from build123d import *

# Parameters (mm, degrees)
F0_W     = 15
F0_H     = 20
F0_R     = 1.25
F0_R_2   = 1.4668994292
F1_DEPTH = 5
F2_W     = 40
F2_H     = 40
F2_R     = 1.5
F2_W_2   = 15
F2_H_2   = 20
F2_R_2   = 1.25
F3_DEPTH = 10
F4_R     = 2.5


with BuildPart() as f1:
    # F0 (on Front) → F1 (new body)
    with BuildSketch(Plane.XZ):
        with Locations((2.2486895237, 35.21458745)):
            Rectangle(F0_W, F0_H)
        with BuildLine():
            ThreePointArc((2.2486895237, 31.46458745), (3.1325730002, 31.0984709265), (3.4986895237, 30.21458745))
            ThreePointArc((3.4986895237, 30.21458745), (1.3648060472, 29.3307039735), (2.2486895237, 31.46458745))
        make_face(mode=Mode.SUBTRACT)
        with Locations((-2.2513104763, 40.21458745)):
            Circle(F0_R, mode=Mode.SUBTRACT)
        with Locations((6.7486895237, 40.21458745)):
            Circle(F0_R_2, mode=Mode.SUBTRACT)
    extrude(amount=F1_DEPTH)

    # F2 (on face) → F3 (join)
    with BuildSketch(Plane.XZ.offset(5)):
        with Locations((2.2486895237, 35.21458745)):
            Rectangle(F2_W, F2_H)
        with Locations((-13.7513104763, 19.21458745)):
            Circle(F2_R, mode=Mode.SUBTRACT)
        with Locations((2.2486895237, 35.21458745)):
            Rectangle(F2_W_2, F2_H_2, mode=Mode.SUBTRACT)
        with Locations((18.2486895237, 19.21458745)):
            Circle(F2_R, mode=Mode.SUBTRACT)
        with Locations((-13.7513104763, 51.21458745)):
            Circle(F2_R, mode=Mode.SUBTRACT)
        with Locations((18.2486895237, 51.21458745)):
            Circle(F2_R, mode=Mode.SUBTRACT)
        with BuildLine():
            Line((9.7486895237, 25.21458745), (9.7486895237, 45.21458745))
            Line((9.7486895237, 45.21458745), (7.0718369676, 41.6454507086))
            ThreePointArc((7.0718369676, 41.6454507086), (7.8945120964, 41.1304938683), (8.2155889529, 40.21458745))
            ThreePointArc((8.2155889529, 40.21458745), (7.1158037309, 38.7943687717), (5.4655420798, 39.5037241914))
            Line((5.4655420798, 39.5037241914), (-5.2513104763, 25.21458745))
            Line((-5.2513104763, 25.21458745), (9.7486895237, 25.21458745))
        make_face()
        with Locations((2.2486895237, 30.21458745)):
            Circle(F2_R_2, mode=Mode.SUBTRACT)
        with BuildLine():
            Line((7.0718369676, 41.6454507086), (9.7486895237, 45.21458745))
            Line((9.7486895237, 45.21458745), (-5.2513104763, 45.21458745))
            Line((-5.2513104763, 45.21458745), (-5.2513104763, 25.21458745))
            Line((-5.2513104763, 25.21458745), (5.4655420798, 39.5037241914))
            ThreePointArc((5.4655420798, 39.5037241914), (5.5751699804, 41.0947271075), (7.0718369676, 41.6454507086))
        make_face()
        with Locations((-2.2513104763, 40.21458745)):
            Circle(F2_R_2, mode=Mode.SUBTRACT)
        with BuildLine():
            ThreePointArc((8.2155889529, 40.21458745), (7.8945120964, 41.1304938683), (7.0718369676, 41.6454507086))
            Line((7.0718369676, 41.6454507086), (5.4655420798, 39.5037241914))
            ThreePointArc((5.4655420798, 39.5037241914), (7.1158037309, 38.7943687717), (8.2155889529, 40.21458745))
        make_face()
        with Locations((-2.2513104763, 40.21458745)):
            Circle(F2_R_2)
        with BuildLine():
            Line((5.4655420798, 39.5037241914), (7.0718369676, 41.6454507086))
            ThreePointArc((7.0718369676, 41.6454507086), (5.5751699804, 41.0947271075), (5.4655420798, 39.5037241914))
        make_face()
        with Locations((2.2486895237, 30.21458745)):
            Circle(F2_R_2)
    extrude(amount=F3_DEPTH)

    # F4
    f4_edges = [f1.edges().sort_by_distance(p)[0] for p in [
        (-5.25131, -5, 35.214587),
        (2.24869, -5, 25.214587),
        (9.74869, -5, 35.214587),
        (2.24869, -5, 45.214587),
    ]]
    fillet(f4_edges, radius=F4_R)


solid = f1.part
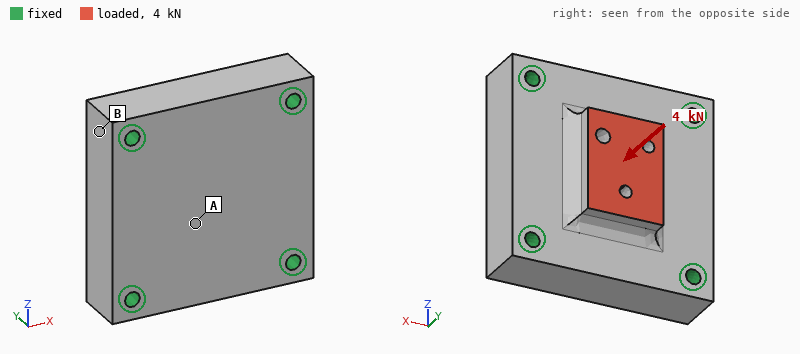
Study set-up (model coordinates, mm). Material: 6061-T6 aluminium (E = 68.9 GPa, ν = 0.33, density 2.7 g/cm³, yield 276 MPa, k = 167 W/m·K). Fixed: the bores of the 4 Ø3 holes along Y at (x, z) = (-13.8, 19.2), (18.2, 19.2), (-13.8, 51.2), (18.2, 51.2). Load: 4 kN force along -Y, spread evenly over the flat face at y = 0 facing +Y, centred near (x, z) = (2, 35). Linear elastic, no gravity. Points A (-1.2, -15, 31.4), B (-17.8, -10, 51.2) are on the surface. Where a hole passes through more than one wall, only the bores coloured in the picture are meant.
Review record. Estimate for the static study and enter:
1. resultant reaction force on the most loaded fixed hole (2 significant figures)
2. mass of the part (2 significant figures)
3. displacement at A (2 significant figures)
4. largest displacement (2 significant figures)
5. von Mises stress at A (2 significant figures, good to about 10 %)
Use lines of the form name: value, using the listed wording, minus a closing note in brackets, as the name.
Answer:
resultant reaction force on the most loaded fixed hole: 1.0 kN
mass of the part: 47 g
displacement at A: 7.9 µm
largest displacement: 9.3 µm
von Mises stress at A: 17 MPa
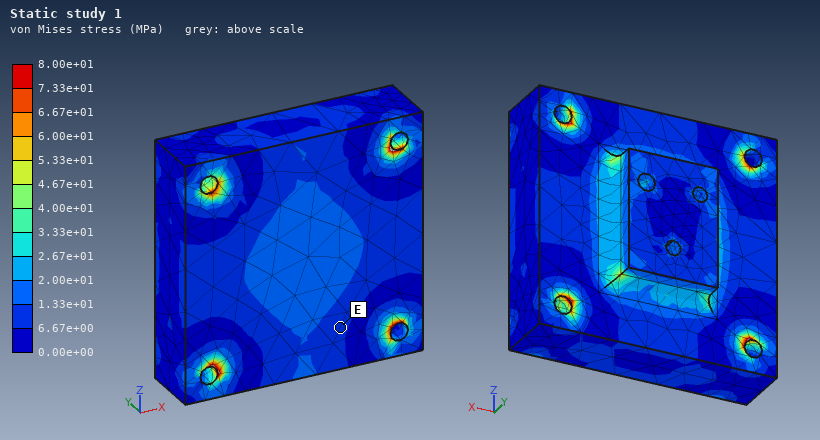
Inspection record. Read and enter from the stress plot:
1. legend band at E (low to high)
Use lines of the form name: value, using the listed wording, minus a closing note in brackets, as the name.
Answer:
legend band at E: 6.67e+00 to 1.33e+01 MPa
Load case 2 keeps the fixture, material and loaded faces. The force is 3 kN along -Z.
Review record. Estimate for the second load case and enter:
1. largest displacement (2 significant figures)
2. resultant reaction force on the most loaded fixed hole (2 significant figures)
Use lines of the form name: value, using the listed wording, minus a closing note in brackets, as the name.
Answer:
largest displacement: 9.1 µm
resultant reaction force on the most loaded fixed hole: 980 N
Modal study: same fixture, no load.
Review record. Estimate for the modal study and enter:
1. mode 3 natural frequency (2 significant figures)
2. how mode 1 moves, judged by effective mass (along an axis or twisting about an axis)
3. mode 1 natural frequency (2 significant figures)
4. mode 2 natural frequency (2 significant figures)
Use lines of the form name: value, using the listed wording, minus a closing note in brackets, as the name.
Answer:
mode 3 natural frequency: 34 kHz
how mode 1 moves, judged by effective mass: along Y
mode 1 natural frequency: 23 kHz
mode 2 natural frequency: 33 kHz
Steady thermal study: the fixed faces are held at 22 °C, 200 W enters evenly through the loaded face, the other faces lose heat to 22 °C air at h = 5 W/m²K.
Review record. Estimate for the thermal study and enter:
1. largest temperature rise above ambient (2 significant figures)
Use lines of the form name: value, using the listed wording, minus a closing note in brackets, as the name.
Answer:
largest temperature rise above ambient: 59 K
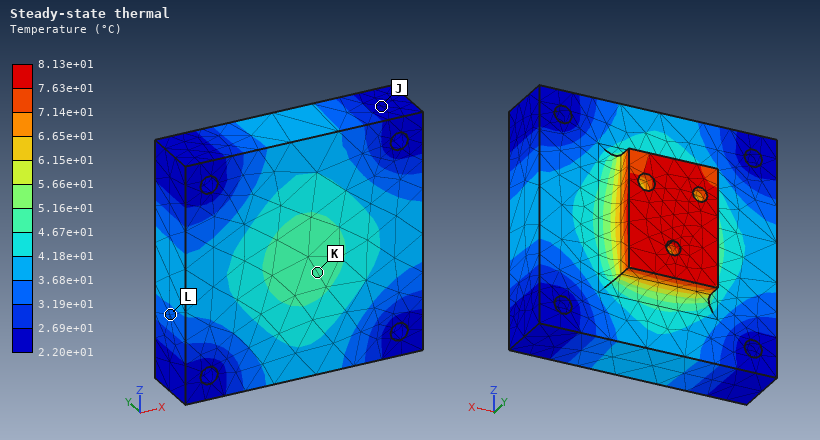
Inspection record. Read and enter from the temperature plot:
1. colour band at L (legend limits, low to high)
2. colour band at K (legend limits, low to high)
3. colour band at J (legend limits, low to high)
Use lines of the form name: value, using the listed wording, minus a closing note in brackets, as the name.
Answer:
colour band at L: 3.19e+01 to 3.68e+01 °C
colour band at K: 4.67e+01 to 5.16e+01 °C
colour band at J: 2.20e+01 to 2.69e+01 °C
